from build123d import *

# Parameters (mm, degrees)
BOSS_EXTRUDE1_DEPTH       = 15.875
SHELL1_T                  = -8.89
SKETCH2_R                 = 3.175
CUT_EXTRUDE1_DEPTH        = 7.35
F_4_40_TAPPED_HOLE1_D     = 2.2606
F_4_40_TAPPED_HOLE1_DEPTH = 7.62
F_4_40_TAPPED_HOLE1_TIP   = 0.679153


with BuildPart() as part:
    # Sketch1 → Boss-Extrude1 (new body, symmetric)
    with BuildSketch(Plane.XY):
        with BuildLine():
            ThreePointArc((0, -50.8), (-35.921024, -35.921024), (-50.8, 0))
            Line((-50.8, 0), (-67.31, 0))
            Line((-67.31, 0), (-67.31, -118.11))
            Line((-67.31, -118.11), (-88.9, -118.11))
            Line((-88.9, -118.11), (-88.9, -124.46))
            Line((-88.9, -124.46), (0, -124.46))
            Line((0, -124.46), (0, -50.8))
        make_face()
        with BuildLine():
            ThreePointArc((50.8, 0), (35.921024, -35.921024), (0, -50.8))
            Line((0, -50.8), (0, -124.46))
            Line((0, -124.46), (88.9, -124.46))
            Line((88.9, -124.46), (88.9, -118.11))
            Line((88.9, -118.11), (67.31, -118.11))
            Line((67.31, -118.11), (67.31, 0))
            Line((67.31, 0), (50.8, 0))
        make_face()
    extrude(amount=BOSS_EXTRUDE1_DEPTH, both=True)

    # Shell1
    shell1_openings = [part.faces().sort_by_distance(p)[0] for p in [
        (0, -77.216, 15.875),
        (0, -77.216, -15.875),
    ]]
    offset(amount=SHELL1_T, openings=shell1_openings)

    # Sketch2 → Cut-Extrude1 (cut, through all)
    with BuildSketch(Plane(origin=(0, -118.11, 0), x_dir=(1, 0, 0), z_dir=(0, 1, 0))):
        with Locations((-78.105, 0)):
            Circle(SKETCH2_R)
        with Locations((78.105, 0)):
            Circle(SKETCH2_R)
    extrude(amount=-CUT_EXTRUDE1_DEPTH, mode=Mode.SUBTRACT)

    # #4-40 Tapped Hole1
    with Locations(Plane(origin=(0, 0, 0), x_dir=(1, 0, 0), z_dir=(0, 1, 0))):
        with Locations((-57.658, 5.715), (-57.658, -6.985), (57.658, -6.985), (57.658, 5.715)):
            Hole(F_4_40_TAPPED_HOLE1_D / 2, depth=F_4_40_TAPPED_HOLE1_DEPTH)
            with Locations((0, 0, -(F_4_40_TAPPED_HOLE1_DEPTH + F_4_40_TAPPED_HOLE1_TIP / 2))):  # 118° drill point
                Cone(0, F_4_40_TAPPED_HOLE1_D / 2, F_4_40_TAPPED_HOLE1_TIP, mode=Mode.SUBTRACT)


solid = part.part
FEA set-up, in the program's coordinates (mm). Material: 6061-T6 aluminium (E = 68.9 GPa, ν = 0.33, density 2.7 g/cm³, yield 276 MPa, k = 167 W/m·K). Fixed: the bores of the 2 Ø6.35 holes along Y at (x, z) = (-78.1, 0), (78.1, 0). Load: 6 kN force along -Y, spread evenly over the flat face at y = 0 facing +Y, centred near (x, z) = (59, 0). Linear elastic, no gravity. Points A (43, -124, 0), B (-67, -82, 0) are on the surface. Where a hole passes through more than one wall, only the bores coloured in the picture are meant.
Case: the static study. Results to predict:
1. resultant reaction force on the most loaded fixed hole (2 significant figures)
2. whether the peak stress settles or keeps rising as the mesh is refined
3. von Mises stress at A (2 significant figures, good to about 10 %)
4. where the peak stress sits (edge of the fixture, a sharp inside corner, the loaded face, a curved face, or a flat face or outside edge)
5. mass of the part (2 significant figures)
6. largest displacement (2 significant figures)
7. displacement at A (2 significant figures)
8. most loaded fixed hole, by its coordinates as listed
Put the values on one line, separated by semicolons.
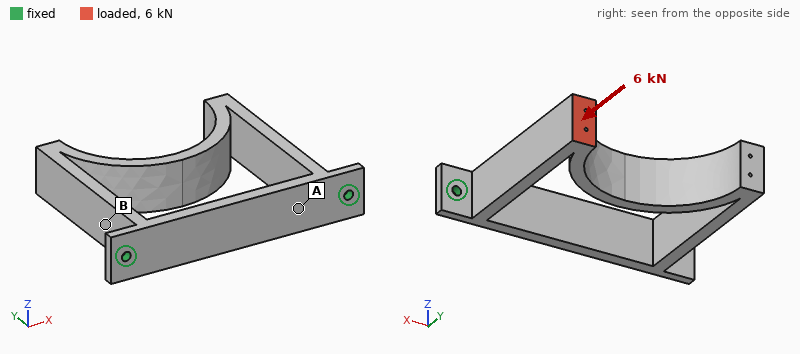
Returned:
5.6 kN; keeps rising; 34 MPa; edge of the fixture; 430 g; 0.40 mm; 0.14 mm; (78.1, 0)
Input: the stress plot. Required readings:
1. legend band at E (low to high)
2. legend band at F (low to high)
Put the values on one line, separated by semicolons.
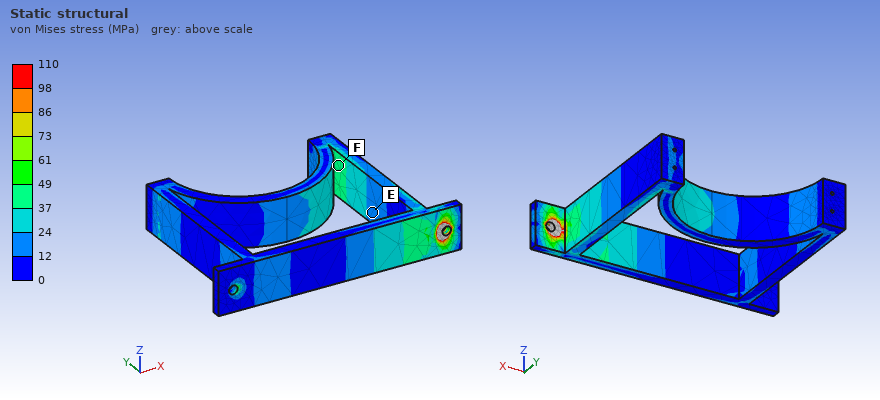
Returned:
12 to 24 MPa; 37 to 49 MPa
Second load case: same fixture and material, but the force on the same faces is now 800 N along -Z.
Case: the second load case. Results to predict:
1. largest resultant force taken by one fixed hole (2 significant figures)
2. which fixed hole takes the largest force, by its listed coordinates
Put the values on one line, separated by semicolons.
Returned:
720 N; (78.1, 0)
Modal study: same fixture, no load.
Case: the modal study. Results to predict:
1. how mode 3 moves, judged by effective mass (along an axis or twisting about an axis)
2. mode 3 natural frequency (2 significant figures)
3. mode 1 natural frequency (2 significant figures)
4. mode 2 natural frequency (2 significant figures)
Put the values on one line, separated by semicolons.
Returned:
twisting about Y; 660 Hz; 390 Hz; 400 Hz
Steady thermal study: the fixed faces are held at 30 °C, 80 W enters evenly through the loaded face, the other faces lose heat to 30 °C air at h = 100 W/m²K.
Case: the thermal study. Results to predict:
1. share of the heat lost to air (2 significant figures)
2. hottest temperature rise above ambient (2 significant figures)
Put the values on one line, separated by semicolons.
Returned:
84 %; 66 K
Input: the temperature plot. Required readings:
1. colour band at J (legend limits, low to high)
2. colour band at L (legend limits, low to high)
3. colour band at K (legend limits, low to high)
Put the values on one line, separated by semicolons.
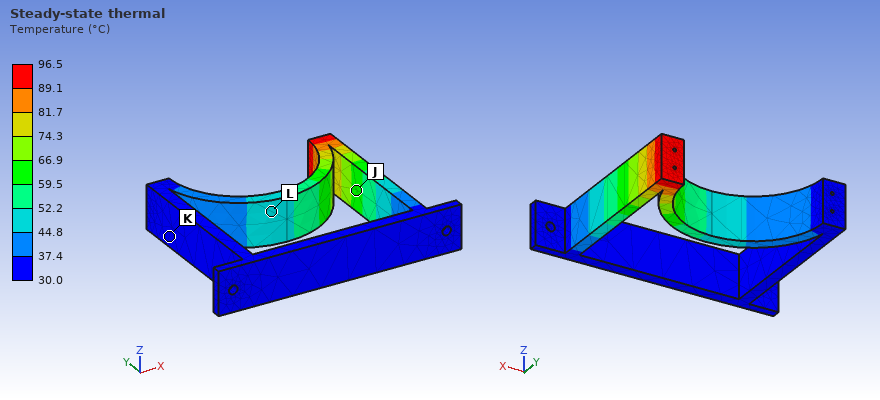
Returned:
59.5 to 66.9 °C; 44.8 to 52.2 °C; 30.0 to 37.4 °C
